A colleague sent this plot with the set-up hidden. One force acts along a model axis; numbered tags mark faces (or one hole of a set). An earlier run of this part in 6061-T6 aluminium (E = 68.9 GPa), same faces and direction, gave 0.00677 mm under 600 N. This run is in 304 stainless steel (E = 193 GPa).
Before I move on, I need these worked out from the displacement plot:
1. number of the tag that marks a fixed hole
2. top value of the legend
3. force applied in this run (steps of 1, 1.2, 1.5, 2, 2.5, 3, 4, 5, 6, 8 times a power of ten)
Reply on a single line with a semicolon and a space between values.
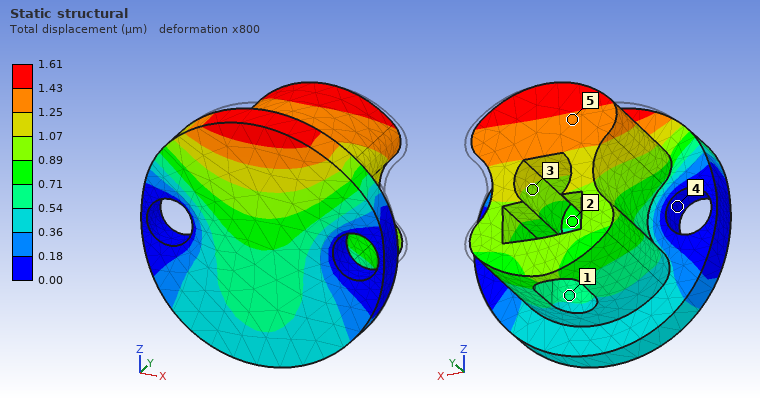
4; 1.61 µm; 400 N
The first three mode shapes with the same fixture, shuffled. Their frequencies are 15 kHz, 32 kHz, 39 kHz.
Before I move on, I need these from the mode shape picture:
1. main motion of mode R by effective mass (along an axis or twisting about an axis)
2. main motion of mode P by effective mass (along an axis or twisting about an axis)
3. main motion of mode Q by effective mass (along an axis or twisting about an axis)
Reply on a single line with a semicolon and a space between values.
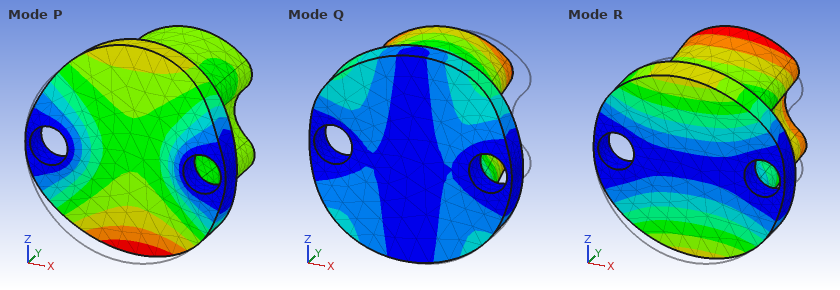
along Z; along Y; along X
